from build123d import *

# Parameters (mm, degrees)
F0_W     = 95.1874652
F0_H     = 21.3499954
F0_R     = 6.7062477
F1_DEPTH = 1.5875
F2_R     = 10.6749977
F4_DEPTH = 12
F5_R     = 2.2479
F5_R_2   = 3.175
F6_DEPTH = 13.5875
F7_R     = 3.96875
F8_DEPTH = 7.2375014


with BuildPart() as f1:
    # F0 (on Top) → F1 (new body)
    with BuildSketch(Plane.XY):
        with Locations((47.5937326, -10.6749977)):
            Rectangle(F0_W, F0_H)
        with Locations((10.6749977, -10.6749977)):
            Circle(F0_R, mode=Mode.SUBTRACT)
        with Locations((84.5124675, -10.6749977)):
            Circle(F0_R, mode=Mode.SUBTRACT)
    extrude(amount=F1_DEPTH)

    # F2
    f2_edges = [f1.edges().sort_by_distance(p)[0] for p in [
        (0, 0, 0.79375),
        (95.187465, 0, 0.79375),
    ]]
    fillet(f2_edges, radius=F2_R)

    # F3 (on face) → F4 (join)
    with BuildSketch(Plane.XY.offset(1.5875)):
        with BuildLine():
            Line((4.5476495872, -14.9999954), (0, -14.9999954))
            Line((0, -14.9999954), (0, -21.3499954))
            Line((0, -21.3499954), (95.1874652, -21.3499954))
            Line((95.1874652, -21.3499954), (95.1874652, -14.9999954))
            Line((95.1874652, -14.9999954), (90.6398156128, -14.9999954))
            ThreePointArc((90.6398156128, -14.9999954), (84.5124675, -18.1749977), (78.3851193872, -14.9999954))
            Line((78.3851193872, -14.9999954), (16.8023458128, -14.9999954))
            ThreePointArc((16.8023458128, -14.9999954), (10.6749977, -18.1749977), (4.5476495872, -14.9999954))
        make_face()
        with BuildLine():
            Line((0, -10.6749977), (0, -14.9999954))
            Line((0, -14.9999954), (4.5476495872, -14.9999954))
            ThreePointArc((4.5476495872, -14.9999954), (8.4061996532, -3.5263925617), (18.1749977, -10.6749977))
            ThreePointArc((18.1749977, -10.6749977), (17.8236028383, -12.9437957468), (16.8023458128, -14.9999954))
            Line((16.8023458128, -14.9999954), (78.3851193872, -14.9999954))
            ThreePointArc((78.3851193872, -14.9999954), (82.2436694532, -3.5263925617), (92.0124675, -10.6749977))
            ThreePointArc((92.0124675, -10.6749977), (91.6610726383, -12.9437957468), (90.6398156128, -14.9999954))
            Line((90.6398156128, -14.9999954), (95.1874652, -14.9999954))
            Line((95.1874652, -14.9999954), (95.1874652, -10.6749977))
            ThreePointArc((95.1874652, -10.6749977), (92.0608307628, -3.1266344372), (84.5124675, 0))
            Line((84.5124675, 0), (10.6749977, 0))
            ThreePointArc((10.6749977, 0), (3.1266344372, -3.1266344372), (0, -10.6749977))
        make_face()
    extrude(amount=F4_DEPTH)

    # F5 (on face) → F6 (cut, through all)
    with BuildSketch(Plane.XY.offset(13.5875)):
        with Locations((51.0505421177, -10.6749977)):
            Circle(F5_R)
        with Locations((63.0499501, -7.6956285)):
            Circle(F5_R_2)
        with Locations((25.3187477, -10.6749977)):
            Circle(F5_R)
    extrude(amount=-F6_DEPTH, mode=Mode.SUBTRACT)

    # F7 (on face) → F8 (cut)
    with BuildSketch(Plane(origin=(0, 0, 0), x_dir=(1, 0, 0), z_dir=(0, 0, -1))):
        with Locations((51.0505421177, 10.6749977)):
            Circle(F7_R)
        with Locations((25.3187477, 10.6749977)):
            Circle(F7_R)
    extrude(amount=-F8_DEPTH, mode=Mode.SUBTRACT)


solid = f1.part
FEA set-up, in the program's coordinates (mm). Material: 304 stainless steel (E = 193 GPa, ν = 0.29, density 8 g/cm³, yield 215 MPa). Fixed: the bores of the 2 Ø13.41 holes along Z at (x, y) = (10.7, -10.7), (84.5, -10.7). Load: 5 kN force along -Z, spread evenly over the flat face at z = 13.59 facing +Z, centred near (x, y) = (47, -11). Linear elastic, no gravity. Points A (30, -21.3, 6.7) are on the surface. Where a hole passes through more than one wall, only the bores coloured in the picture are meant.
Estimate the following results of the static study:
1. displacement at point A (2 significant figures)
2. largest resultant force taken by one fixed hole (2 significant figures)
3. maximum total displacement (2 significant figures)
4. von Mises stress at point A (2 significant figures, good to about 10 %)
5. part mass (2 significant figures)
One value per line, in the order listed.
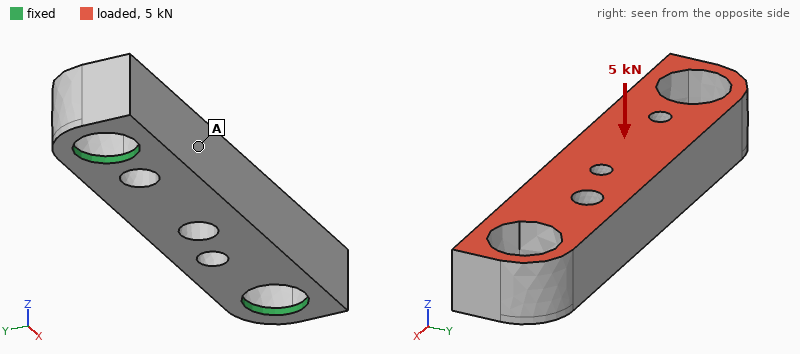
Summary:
7.8 µm
3.1 kN
12 µm
17 MPa
170 g
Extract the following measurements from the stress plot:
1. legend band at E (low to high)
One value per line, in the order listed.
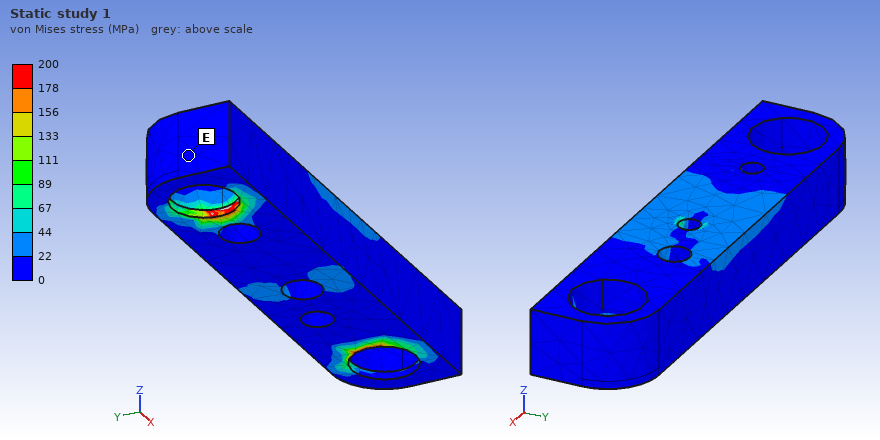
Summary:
0 to 22 MPa
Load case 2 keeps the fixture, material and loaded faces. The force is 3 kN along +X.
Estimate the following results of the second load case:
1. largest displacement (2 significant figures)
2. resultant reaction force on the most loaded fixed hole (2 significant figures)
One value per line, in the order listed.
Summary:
3.0 µm
1.6 kN
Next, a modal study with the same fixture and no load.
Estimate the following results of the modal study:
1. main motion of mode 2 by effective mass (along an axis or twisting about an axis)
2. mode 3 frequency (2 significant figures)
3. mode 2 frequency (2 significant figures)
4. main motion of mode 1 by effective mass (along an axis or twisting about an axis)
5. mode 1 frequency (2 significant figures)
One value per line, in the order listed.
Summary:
along Z
13 kHz
9000 Hz
along Y
8200 Hz
